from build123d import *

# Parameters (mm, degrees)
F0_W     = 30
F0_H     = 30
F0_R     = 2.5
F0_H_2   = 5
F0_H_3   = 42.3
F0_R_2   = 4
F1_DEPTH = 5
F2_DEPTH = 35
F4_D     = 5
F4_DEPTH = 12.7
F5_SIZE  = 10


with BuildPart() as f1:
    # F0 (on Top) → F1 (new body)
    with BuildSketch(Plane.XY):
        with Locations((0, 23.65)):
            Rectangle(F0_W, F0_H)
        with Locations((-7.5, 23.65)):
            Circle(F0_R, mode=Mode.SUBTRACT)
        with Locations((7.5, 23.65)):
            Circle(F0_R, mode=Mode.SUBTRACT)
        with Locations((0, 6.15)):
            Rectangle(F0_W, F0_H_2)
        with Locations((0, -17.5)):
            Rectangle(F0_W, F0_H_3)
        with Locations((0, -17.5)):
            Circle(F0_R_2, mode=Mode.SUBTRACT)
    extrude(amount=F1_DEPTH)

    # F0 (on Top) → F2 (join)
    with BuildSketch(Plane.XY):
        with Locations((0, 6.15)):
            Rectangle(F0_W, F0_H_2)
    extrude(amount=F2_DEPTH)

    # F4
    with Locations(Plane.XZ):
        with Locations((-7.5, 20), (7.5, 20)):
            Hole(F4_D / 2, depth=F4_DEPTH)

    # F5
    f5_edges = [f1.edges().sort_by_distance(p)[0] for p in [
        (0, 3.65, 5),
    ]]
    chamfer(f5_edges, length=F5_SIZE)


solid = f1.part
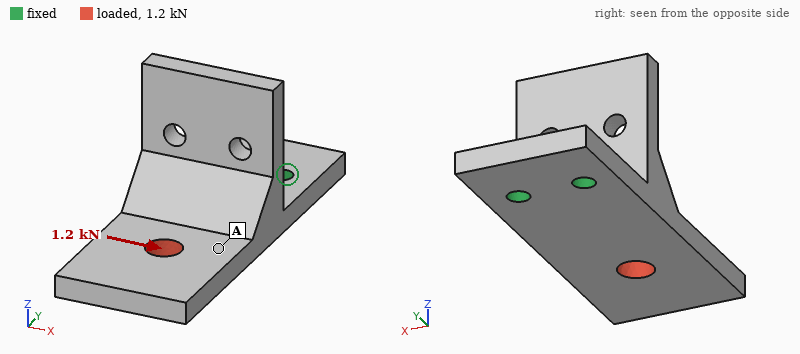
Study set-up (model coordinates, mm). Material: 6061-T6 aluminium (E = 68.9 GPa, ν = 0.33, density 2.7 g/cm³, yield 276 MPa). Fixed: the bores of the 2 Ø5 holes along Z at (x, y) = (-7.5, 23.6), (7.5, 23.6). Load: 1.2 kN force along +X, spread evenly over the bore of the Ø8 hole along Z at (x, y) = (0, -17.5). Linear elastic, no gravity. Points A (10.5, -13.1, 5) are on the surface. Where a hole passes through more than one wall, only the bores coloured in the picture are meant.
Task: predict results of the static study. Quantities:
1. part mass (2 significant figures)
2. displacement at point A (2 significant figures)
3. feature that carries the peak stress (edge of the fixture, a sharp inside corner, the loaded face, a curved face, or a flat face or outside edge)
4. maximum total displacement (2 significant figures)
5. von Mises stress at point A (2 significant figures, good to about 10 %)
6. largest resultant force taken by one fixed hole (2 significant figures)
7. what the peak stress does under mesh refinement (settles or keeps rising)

46 g
47 µm
edge of the fixture
88 µm
14 MPa
2.8 kN
keeps rising
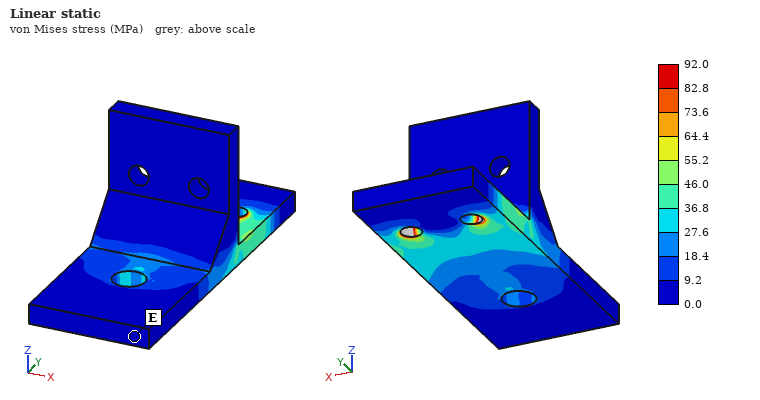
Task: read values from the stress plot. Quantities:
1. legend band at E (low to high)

0.0 to 9.2 MPa
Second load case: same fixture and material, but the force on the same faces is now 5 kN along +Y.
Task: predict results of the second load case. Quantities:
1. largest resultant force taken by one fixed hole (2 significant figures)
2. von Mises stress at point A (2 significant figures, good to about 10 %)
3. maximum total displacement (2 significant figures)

2.5 kN
26 MPa
47 µm
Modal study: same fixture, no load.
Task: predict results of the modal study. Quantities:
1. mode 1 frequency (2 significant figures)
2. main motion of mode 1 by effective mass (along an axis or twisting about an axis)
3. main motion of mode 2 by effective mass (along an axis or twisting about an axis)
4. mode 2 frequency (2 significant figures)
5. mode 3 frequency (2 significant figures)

1100 Hz
along Z
along X
3700 Hz
4700 Hz
